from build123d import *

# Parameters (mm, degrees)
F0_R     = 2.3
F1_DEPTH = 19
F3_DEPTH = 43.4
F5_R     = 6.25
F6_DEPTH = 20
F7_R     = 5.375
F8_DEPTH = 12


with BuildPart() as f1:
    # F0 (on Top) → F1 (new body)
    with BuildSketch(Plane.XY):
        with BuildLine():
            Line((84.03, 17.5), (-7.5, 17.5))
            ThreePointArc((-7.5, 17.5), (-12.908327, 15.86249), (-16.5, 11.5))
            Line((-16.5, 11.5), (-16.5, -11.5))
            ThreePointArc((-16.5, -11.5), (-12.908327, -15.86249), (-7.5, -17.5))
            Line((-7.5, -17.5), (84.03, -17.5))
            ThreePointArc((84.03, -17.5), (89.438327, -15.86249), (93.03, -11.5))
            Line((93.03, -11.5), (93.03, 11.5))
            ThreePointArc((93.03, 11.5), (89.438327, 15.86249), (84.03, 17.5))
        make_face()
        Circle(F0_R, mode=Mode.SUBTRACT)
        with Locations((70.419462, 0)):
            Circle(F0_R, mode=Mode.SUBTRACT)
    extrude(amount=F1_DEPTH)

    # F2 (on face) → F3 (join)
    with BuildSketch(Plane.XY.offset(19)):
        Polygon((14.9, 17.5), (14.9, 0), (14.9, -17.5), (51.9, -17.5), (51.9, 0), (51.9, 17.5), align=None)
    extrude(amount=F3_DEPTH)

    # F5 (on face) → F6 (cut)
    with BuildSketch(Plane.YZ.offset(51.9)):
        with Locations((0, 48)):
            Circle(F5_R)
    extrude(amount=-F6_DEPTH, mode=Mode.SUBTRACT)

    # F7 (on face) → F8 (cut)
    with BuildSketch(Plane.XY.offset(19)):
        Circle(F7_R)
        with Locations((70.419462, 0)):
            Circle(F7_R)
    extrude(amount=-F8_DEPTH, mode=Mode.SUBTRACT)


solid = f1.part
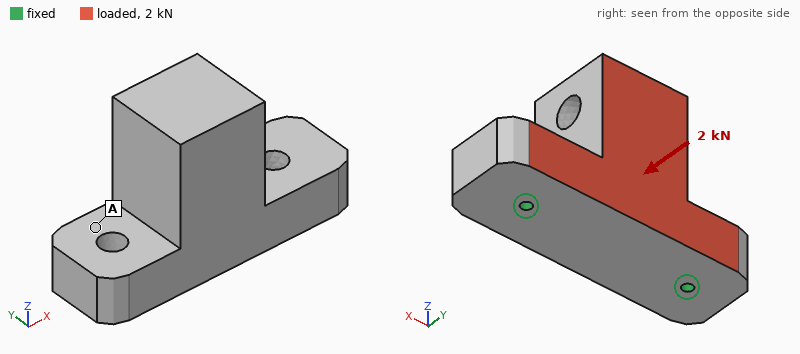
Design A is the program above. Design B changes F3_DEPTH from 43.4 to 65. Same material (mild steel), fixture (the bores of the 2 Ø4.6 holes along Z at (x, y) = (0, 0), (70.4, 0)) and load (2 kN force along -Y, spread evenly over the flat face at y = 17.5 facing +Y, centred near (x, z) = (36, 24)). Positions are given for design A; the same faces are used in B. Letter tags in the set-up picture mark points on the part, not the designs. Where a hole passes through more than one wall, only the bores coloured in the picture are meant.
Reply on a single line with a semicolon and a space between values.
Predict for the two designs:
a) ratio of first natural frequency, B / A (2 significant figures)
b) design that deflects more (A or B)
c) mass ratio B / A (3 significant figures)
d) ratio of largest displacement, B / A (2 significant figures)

0.64; B; 1.23; 2.0
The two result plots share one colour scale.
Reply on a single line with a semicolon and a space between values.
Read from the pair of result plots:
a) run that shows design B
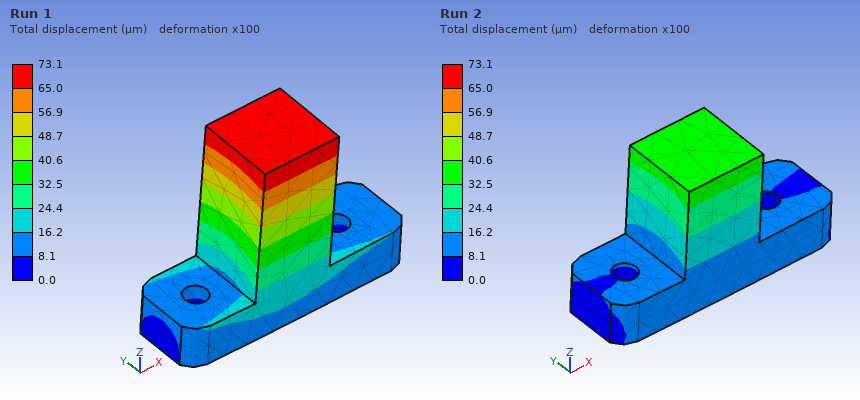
Run 1
